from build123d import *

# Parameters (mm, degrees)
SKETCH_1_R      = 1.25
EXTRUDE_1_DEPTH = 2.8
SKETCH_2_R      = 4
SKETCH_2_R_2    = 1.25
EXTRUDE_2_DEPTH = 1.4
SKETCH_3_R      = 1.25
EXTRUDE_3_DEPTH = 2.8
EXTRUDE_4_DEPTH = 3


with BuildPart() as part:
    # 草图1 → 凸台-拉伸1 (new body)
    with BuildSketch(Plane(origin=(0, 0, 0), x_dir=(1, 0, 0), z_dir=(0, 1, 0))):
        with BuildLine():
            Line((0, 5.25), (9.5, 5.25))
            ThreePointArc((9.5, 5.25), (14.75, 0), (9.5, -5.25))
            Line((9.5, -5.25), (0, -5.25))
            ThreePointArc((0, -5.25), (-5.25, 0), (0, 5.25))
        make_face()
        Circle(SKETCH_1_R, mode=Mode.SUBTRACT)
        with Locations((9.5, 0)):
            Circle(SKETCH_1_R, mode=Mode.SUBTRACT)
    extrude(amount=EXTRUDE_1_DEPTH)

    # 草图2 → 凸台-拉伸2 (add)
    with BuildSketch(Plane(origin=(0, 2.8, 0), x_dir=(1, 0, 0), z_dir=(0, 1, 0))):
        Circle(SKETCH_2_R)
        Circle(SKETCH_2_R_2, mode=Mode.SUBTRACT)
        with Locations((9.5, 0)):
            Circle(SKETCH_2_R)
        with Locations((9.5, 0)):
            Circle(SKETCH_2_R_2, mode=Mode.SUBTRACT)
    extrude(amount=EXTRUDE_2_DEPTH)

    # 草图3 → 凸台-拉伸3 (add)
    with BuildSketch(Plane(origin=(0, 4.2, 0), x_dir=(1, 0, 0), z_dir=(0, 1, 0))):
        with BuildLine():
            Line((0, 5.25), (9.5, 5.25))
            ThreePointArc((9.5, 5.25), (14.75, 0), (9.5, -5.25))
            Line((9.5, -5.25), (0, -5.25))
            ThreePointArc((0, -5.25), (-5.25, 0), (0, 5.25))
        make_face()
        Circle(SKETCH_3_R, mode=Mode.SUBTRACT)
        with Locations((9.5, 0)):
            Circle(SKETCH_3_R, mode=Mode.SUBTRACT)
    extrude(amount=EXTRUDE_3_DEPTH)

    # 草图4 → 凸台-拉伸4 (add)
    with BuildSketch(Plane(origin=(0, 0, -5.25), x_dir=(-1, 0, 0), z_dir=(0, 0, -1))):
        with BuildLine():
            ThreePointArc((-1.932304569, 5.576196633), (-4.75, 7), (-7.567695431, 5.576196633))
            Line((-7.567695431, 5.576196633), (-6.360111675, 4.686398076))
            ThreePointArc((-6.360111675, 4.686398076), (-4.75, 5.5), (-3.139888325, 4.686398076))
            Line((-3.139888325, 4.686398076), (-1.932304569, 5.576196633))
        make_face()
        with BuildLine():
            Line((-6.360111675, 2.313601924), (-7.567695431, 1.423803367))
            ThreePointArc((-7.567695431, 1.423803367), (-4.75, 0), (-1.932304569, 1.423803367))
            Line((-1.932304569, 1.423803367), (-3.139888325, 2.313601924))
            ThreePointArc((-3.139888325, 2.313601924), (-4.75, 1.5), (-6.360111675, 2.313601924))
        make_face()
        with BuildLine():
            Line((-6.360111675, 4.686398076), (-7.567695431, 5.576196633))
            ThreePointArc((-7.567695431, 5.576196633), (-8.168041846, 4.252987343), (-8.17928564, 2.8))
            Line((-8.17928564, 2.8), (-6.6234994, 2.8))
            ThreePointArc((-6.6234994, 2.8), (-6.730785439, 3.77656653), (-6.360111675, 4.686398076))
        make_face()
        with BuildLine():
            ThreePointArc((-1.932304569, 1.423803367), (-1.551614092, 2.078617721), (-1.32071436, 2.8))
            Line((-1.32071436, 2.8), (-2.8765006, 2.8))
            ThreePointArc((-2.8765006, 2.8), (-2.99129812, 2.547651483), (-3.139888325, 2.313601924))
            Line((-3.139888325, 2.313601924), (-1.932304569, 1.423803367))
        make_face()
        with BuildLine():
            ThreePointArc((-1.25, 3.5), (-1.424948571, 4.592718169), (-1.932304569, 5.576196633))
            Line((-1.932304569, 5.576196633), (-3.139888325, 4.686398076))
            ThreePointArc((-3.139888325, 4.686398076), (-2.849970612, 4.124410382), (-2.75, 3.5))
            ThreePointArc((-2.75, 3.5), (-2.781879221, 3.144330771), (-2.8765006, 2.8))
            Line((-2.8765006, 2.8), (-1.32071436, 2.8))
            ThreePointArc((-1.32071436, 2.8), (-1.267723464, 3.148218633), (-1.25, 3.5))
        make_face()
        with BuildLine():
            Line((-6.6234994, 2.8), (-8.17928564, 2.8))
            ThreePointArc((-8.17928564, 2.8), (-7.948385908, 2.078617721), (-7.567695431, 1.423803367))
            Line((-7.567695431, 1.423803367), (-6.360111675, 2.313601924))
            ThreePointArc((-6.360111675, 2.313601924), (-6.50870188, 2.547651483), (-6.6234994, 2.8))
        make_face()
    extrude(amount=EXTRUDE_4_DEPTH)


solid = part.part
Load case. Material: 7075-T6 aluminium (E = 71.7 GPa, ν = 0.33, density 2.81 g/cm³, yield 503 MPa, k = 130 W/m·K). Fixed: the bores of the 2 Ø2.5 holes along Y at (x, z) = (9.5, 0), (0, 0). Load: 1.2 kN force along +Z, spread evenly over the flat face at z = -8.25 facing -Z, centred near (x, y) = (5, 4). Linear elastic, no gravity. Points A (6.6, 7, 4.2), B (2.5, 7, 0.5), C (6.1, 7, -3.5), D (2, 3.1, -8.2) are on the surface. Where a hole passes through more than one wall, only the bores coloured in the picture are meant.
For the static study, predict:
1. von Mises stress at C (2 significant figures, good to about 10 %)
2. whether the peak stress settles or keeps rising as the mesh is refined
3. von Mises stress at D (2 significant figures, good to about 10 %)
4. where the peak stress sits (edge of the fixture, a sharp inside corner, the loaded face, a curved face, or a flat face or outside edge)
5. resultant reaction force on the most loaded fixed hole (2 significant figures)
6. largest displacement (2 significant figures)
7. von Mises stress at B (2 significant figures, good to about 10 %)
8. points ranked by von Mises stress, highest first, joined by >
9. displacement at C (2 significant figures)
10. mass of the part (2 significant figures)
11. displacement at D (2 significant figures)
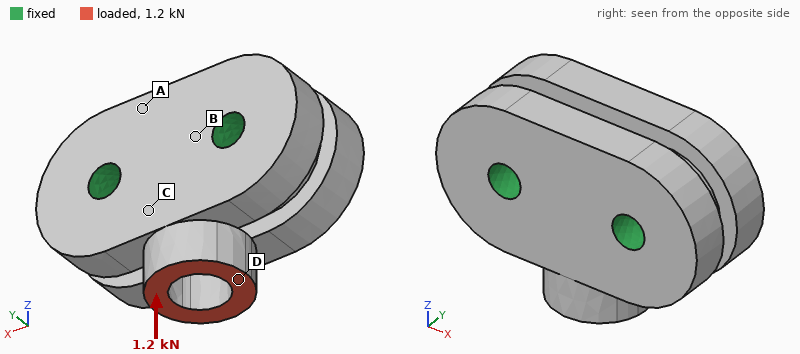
25 MPa
keeps rising
45 MPa
a sharp inside corner
640 N
4.5 µm
14 MPa
D > C > B > A
1.8 µm
3.4 g
4.3 µm
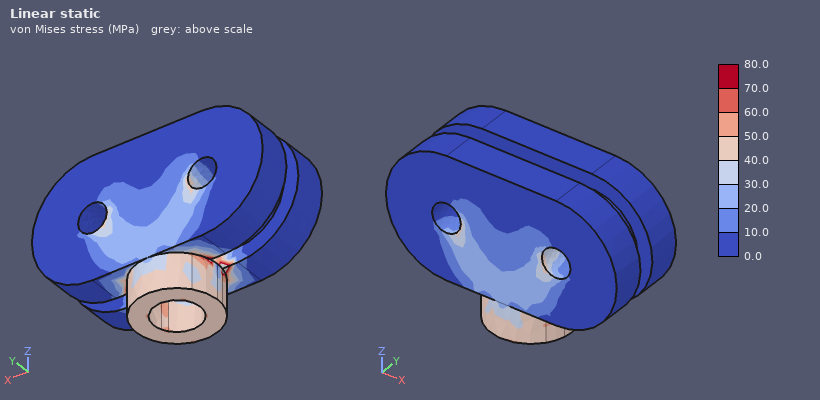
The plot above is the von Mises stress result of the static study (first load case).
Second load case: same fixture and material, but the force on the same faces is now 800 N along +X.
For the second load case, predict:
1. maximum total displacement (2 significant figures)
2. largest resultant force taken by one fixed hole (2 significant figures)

16 µm
730 N
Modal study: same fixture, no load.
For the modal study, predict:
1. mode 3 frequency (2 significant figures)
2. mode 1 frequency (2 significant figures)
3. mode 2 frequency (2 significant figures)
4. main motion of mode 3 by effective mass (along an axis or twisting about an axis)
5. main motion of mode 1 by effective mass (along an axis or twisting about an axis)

110 kHz
73 kHz
100 kHz
along Y
along Y
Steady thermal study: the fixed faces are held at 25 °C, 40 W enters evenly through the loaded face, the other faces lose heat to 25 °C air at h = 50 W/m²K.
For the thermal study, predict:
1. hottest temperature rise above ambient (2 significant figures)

65 K
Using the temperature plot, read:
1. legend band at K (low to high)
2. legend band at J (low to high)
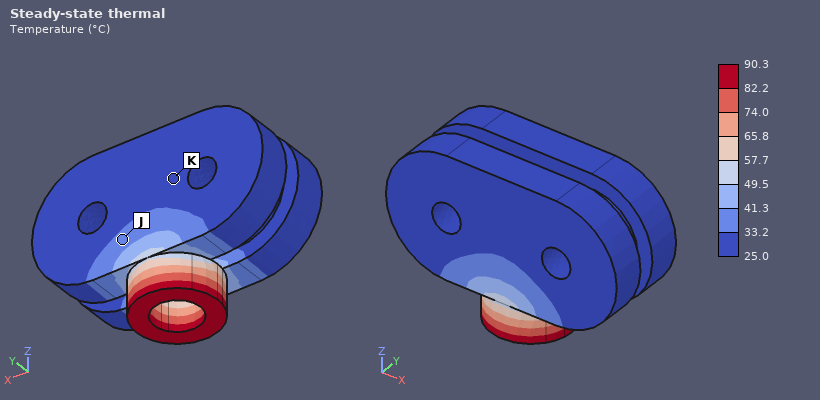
25.0 to 33.2 °C
33.2 to 41.3 °C
